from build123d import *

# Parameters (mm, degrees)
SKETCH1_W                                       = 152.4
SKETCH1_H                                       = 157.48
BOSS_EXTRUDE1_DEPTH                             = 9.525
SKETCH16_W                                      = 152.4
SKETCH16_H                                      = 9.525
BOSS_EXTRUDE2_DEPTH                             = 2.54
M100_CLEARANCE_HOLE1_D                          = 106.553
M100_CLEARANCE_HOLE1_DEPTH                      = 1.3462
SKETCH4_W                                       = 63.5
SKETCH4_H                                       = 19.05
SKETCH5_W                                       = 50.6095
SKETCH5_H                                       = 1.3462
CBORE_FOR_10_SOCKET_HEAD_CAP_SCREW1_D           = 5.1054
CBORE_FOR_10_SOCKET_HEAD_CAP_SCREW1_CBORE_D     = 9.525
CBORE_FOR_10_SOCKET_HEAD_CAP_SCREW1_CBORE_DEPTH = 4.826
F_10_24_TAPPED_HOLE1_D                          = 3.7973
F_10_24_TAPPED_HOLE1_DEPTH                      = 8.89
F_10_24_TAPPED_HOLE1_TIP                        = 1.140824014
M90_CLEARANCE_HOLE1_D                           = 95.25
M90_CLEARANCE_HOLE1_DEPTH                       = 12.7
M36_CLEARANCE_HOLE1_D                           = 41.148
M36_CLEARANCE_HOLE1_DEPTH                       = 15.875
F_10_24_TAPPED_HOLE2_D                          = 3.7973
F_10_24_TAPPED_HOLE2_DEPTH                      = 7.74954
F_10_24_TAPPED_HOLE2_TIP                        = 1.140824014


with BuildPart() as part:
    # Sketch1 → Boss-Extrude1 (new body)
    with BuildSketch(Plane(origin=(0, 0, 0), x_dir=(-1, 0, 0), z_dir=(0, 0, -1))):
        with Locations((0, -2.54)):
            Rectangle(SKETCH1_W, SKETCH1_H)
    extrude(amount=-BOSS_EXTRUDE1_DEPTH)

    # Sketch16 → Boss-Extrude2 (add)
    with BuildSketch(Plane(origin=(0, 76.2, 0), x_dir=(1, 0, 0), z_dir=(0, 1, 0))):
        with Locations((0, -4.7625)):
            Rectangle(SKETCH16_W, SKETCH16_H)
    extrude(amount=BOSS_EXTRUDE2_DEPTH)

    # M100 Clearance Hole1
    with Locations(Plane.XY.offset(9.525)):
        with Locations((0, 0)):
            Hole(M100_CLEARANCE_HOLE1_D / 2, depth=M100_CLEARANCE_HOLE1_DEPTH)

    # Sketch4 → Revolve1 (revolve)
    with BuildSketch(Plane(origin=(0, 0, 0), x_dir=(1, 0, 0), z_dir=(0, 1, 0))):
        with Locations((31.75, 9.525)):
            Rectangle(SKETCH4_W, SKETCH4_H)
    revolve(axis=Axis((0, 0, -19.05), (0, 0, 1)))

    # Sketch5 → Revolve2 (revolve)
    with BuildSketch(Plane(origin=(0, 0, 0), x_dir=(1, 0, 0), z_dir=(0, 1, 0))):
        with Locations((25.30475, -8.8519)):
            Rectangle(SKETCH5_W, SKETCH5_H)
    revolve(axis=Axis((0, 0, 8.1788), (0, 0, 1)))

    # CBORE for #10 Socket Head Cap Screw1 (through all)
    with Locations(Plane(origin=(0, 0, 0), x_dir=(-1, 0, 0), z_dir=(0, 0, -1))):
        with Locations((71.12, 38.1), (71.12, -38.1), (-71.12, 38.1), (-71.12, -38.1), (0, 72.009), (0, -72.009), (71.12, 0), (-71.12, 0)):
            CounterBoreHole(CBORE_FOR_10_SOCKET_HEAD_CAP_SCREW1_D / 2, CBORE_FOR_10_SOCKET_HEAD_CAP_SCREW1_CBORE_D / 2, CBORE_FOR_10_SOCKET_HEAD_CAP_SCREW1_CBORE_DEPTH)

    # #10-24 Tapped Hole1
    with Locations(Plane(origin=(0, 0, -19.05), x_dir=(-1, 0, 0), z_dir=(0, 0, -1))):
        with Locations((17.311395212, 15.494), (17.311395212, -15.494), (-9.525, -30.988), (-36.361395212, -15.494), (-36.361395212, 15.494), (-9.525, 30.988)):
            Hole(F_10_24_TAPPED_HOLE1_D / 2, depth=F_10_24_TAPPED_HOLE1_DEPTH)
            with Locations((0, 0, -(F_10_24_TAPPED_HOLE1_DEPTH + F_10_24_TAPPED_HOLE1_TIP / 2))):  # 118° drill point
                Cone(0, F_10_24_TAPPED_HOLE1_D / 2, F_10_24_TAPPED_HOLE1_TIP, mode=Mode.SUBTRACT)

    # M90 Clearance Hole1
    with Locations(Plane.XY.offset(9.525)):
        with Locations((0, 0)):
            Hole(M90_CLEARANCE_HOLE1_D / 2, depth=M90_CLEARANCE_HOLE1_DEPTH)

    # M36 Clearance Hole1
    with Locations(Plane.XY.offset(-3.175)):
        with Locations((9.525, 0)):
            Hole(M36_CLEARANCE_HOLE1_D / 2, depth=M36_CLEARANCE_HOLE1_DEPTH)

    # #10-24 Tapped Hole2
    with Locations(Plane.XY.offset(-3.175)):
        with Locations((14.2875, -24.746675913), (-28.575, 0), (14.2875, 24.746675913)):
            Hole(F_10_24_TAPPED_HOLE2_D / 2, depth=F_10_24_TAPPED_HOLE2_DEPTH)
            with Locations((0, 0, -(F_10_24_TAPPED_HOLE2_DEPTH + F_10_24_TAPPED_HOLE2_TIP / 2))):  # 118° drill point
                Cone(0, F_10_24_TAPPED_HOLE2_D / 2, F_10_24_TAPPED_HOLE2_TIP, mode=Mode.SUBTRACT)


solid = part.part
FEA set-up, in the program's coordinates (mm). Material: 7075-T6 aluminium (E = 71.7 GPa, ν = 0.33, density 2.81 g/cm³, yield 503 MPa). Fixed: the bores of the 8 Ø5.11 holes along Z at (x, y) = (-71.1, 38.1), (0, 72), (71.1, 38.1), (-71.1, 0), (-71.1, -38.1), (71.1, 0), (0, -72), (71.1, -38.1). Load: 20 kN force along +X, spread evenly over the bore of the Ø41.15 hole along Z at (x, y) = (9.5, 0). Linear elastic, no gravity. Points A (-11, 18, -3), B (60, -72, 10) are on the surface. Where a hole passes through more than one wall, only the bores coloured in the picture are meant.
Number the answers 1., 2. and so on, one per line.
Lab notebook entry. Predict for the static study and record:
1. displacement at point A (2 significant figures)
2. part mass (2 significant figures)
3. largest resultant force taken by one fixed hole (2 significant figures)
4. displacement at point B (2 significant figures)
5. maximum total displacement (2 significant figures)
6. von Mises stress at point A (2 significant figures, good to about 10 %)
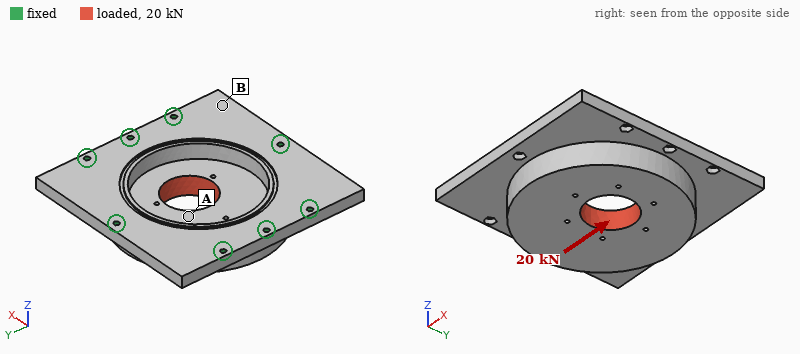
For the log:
1. 14 µm
2. 1.0 kg
3. 2.9 kN
4. 6.8 µm
5. 20 µm
6. 12 MPa
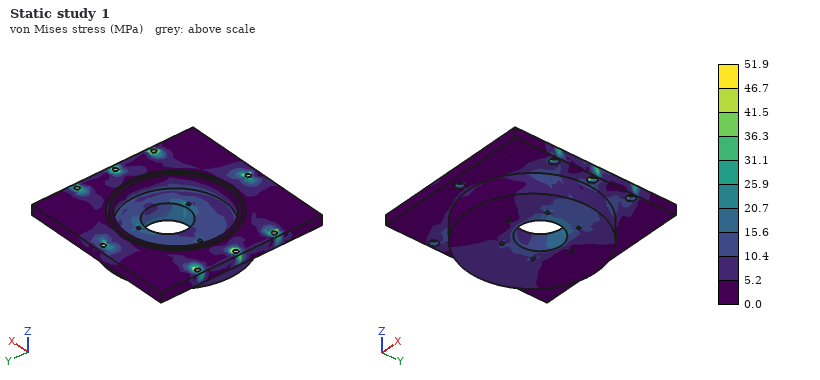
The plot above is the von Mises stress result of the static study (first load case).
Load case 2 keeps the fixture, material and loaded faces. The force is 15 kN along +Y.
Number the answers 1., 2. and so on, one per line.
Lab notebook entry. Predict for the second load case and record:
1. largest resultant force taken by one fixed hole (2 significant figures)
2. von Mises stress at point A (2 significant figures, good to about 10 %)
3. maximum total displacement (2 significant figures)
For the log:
1. 3.2 kN
2. 9.4 MPa
3. 14 µm
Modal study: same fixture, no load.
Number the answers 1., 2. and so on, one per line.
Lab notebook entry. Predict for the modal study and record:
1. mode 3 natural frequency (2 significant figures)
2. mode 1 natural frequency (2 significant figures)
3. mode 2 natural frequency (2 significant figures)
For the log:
1. 4900 Hz
2. 4700 Hz
3. 4800 Hz
